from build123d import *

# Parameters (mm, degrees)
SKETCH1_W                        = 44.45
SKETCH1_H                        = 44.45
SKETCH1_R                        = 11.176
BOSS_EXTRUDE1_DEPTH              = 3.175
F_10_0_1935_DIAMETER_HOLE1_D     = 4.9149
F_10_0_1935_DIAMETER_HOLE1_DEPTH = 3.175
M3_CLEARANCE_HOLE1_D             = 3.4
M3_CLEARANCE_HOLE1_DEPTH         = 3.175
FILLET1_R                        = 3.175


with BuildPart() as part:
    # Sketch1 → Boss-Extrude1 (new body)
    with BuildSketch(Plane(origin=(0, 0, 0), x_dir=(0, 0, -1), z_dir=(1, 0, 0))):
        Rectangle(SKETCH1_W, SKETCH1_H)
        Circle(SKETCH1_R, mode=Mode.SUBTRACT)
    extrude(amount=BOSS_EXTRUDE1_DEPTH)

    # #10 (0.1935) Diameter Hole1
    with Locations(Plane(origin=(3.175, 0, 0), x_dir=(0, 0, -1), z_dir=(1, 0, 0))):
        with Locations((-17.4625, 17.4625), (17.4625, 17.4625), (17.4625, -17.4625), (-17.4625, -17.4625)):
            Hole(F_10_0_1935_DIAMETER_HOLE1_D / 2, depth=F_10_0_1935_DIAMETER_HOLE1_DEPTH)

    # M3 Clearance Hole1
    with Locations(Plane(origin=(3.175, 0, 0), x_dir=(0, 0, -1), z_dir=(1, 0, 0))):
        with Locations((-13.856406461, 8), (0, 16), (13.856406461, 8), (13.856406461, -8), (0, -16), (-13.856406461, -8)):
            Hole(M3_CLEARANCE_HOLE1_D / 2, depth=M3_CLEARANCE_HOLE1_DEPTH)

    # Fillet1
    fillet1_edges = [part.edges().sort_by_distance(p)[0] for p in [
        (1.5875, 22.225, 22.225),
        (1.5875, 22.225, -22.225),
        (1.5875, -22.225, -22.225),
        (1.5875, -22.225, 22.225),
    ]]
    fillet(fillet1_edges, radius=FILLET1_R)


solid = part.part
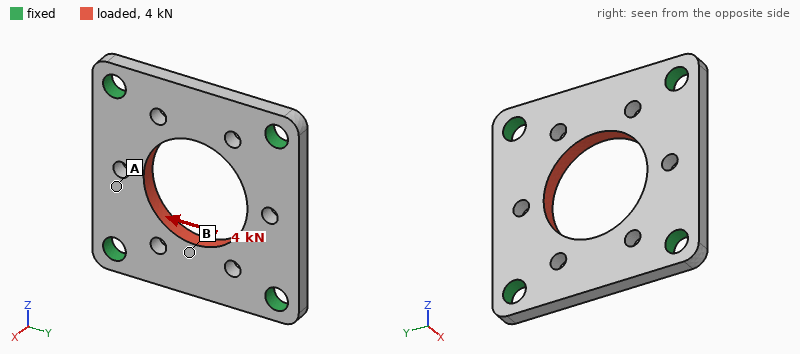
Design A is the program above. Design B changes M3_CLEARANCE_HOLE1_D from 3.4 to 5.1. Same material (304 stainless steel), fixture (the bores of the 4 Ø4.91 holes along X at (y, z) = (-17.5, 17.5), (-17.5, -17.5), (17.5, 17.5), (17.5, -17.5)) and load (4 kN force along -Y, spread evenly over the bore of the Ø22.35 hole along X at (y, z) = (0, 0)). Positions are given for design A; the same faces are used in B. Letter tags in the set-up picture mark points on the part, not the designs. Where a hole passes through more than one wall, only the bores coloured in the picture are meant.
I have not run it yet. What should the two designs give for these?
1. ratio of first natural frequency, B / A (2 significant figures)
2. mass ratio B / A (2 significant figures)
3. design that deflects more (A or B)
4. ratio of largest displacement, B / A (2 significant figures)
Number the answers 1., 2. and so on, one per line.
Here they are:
1. 1.0
2. 0.95
3. B
4. 1.2
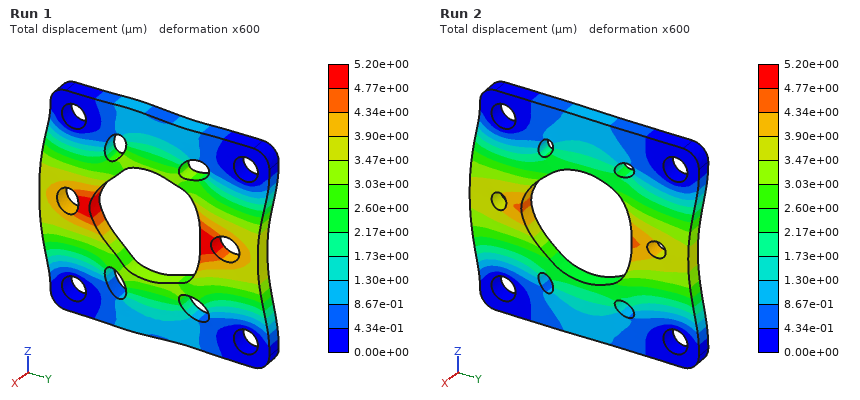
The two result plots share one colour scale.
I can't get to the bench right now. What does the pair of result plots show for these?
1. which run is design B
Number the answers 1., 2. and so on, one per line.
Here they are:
1. Run 1
